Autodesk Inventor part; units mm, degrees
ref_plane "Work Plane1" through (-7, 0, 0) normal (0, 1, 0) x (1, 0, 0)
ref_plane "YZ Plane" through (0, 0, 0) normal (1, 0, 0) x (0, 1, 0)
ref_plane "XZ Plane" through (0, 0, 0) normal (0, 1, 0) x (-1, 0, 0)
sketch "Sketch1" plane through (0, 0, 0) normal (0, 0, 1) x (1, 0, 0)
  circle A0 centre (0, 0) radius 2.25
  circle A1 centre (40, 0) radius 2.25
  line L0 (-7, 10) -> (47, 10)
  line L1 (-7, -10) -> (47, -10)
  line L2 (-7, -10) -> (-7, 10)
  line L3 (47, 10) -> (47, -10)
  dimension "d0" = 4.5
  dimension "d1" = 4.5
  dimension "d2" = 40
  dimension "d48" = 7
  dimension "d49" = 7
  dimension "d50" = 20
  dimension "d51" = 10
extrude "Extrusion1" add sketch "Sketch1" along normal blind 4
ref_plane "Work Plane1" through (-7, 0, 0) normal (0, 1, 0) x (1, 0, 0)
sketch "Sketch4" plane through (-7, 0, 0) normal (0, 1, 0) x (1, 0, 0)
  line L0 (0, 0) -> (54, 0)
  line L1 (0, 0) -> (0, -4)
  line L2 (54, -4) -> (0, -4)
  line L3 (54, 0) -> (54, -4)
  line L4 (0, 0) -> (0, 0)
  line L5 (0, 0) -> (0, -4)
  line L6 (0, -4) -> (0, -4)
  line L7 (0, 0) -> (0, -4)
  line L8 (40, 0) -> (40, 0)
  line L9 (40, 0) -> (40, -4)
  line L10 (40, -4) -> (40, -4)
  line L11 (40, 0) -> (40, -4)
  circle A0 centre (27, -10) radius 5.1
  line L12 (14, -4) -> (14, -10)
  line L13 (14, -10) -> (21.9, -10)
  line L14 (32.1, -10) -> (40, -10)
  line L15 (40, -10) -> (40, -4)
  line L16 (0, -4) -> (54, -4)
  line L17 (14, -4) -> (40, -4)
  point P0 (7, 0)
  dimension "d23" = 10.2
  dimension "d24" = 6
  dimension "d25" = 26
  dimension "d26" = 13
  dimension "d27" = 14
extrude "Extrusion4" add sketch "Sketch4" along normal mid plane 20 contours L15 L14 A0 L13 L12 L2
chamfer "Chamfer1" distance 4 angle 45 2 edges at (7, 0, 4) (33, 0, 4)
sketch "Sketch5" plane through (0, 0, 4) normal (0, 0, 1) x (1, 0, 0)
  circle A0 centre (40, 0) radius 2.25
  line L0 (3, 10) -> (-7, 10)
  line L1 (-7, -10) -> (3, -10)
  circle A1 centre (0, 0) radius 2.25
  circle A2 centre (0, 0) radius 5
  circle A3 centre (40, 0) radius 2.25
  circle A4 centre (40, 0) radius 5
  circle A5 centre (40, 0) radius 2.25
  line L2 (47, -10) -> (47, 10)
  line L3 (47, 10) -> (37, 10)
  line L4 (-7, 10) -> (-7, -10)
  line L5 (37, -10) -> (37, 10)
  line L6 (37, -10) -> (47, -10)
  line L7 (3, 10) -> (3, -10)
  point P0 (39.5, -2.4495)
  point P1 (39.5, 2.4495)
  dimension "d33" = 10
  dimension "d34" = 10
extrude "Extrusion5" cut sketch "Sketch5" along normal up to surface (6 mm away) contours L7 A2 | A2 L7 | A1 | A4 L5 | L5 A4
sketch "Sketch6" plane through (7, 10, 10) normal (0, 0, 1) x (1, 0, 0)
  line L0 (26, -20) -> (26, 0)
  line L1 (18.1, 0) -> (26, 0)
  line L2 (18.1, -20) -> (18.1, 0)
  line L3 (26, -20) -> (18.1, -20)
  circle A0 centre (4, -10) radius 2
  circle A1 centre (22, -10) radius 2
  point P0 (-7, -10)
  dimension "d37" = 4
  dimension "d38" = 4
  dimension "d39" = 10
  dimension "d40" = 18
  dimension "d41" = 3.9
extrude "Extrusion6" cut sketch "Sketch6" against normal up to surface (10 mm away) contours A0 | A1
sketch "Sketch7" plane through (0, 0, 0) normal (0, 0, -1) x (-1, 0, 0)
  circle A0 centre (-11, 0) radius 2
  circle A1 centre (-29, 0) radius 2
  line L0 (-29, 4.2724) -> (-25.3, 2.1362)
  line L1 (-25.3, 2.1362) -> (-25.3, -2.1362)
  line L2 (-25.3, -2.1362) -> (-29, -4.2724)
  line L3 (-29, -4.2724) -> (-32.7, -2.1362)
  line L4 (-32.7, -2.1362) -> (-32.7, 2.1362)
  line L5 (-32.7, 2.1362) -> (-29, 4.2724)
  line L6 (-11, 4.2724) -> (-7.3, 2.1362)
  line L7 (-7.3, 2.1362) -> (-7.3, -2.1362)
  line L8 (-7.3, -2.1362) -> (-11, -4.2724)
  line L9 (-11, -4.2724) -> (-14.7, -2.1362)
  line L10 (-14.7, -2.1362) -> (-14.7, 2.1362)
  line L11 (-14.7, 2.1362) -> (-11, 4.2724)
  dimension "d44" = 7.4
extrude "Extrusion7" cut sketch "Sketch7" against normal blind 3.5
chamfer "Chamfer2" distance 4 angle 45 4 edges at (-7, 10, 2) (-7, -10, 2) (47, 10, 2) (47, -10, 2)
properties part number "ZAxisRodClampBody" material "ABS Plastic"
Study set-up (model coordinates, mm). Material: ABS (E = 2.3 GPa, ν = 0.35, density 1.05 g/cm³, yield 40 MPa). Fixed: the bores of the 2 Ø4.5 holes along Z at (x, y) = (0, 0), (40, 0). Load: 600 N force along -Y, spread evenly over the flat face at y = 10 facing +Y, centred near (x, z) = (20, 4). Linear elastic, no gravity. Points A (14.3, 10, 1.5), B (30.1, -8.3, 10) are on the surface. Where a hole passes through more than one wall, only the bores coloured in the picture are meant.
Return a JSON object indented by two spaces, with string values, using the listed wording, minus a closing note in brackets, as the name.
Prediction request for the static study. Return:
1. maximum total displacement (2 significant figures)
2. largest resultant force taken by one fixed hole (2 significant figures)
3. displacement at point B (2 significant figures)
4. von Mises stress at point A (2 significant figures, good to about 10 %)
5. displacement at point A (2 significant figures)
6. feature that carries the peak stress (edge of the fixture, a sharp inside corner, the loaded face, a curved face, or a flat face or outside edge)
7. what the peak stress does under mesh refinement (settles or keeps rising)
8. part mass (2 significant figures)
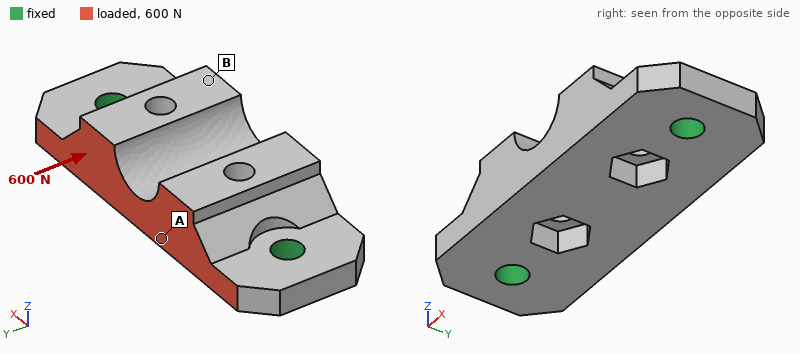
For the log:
{
  "maximum total displacement": "0.15 mm",
  "largest resultant force taken by one fixed hole": "300 N",
  "displacement at point B": "0.12 mm",
  "von Mises stress at point A": "6.4 MPa",
  "displacement at point A": "0.098 mm",
  "feature that carries the peak stress": "edge of the fixture",
  "what the peak stress does under mesh refinement": "keeps rising",
  "part mass": "6.5 g"
}
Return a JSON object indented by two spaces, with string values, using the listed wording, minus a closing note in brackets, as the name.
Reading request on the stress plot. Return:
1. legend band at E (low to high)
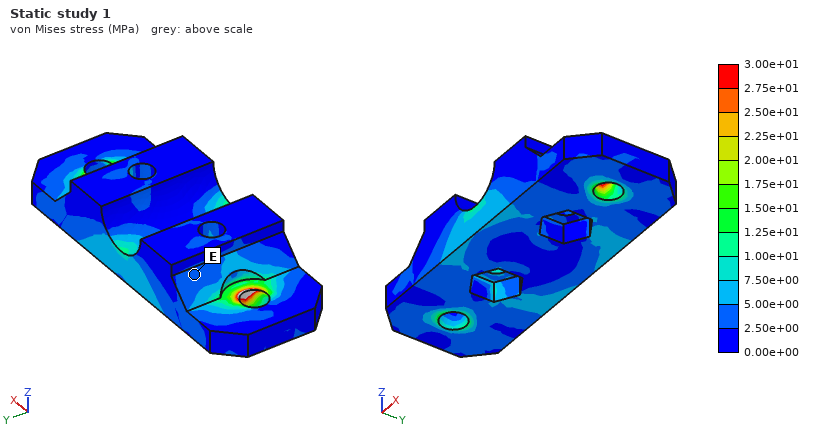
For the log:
{
  "legend band at E": "2.50e+00 to 5.00e+00 MPa"
}
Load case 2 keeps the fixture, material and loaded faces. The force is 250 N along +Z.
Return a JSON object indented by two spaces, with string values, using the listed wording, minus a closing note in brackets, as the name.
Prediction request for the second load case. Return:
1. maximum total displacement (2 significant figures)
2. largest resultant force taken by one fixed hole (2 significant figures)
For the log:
{
  "maximum total displacement": "0.32 mm",
  "largest resultant force taken by one fixed hole": "150 N"
}
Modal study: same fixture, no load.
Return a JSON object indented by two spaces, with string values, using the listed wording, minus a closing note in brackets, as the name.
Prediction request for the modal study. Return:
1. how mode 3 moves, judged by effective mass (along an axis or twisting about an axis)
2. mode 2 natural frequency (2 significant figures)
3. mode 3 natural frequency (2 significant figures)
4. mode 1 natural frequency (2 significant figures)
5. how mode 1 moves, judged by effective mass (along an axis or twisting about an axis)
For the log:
{
  "how mode 3 moves, judged by effective mass": "along Y",
  "mode 2 natural frequency": "3700 Hz",
  "mode 3 natural frequency": "6100 Hz",
  "mode 1 natural frequency": "3500 Hz",
  "how mode 1 moves, judged by effective mass": "along Z"
}
